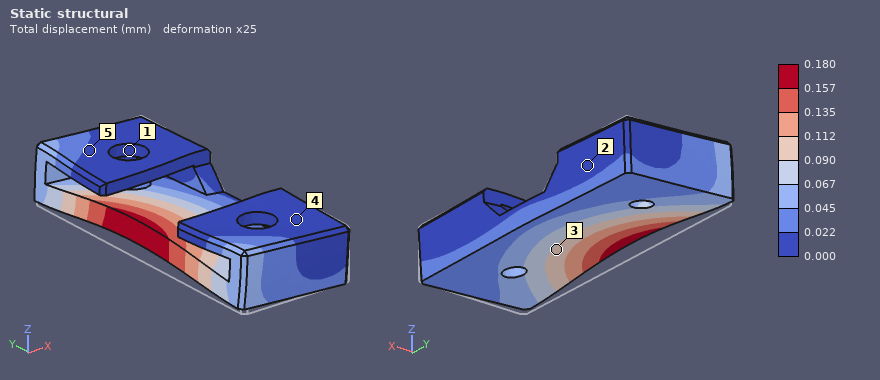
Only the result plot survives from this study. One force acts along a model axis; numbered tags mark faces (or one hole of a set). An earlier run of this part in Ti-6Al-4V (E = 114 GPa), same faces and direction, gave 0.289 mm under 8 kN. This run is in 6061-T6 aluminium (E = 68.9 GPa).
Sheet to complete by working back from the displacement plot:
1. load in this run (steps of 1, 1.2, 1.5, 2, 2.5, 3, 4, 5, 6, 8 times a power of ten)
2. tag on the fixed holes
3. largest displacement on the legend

3 kN
1
0.180 mm
